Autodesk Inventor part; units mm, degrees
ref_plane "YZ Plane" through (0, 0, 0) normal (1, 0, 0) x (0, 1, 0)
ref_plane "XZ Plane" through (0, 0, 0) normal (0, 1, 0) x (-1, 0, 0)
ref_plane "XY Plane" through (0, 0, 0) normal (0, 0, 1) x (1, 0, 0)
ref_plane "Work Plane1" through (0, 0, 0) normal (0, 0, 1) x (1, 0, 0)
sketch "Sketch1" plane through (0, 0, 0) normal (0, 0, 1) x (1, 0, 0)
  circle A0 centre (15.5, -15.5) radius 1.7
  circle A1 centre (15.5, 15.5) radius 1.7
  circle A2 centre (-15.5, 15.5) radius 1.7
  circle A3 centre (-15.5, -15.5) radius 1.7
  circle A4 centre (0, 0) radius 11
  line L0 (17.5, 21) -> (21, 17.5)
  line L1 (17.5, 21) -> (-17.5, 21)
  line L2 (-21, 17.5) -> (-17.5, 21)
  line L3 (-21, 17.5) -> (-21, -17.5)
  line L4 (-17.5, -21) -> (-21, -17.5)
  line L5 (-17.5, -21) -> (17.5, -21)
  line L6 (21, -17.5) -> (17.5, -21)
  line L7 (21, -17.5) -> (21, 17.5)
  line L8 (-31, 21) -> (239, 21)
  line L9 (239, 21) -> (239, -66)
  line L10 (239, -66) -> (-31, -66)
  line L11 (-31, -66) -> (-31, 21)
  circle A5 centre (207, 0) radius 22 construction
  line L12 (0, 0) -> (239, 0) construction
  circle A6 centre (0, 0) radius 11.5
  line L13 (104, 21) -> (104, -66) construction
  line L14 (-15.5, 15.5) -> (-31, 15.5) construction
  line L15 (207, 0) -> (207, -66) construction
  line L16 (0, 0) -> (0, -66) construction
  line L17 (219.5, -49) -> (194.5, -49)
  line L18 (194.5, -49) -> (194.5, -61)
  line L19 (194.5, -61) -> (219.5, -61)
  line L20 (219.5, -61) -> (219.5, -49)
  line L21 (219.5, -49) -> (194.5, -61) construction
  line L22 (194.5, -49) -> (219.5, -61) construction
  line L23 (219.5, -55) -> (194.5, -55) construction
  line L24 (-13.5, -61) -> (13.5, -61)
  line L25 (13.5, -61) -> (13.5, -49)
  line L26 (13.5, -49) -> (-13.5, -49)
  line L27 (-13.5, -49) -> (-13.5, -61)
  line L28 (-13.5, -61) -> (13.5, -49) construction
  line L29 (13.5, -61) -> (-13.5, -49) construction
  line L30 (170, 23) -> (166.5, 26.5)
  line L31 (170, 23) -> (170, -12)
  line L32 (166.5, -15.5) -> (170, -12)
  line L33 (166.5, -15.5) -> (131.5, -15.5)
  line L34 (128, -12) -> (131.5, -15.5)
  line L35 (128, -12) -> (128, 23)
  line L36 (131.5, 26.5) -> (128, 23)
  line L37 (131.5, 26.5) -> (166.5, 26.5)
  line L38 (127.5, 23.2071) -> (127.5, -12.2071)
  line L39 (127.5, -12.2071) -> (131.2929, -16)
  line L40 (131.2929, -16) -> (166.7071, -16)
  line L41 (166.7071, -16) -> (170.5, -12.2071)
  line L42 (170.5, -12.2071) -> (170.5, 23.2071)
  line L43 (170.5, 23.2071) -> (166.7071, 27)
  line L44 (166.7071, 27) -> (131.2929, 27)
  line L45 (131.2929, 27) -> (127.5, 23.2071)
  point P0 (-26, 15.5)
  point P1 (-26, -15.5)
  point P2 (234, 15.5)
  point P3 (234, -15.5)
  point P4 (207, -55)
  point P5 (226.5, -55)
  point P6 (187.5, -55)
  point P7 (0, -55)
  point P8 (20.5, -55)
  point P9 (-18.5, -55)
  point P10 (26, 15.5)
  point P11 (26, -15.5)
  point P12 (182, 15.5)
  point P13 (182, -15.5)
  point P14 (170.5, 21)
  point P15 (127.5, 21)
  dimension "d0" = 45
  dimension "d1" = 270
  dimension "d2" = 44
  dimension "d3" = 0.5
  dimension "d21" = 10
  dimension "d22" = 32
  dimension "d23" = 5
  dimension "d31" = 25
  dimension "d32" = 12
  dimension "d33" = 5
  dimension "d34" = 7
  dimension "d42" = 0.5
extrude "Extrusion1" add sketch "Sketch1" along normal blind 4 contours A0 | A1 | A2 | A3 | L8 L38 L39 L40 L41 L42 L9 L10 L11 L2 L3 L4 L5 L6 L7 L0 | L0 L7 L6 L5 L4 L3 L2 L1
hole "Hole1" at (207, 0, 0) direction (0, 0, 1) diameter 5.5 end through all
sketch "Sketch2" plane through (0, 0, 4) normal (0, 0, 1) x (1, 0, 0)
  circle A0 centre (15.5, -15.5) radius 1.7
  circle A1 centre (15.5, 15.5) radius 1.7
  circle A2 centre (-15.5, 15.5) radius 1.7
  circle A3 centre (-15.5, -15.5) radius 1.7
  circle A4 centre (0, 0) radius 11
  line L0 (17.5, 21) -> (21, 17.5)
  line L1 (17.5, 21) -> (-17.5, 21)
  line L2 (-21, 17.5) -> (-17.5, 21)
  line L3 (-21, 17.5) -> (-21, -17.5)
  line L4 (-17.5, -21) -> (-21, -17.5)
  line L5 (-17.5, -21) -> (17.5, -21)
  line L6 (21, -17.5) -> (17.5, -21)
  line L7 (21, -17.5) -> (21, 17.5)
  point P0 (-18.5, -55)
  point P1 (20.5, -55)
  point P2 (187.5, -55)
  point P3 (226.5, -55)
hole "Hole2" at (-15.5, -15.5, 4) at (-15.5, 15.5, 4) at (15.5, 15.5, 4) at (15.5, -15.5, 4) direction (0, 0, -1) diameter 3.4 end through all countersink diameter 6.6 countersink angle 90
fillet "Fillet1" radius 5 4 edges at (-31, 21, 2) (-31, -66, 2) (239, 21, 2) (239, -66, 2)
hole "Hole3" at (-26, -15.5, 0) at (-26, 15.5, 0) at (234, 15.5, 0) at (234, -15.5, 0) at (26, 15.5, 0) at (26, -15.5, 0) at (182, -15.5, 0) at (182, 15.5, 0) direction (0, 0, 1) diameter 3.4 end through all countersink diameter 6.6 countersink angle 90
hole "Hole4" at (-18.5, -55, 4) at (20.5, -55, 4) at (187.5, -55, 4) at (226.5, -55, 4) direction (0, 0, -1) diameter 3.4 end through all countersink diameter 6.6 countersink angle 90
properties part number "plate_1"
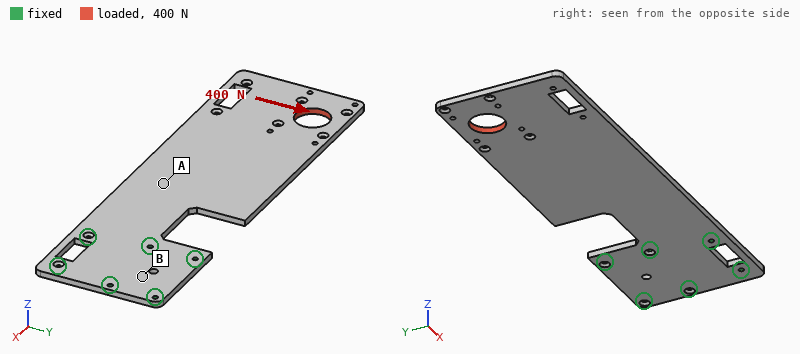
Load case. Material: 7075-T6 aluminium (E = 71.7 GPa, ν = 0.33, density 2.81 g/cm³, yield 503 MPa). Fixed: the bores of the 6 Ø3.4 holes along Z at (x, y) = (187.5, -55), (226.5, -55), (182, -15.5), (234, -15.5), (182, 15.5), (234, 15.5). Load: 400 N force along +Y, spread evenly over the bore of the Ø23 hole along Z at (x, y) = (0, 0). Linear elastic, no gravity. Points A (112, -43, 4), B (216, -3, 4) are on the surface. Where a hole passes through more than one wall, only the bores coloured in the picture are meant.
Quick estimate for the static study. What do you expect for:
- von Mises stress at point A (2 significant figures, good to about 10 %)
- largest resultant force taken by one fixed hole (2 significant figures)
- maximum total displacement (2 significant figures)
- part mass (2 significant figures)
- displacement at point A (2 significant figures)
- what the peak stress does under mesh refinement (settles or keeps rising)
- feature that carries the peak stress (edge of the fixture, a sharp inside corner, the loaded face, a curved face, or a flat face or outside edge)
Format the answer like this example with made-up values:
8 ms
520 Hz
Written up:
10 MPa
1.4 kN
0.33 mm
230 g
0.073 mm
keeps rising
edge of the fixture
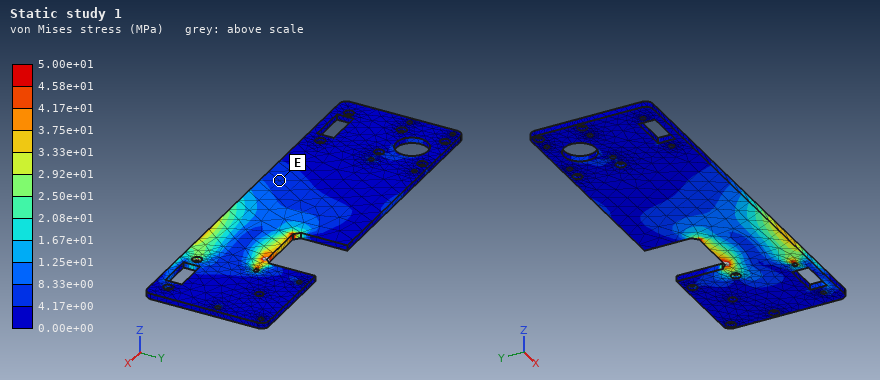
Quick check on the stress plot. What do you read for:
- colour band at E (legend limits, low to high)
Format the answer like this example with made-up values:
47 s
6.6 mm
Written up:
4.17e+00 to 8.33e+00 MPa
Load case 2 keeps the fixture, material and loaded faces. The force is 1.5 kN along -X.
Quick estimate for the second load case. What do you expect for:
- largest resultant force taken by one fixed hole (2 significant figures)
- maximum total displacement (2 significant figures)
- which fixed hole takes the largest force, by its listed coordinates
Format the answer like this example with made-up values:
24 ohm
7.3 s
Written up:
1.5 kN
0.33 mm
(182, -15.5)
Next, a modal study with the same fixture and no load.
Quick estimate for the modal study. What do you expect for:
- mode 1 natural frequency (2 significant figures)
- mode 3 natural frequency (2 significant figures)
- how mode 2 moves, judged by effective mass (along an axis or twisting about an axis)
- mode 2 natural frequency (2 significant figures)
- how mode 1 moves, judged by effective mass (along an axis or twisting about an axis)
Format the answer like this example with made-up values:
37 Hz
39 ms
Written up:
58 Hz
400 Hz
twisting about X
290 Hz
along Z
